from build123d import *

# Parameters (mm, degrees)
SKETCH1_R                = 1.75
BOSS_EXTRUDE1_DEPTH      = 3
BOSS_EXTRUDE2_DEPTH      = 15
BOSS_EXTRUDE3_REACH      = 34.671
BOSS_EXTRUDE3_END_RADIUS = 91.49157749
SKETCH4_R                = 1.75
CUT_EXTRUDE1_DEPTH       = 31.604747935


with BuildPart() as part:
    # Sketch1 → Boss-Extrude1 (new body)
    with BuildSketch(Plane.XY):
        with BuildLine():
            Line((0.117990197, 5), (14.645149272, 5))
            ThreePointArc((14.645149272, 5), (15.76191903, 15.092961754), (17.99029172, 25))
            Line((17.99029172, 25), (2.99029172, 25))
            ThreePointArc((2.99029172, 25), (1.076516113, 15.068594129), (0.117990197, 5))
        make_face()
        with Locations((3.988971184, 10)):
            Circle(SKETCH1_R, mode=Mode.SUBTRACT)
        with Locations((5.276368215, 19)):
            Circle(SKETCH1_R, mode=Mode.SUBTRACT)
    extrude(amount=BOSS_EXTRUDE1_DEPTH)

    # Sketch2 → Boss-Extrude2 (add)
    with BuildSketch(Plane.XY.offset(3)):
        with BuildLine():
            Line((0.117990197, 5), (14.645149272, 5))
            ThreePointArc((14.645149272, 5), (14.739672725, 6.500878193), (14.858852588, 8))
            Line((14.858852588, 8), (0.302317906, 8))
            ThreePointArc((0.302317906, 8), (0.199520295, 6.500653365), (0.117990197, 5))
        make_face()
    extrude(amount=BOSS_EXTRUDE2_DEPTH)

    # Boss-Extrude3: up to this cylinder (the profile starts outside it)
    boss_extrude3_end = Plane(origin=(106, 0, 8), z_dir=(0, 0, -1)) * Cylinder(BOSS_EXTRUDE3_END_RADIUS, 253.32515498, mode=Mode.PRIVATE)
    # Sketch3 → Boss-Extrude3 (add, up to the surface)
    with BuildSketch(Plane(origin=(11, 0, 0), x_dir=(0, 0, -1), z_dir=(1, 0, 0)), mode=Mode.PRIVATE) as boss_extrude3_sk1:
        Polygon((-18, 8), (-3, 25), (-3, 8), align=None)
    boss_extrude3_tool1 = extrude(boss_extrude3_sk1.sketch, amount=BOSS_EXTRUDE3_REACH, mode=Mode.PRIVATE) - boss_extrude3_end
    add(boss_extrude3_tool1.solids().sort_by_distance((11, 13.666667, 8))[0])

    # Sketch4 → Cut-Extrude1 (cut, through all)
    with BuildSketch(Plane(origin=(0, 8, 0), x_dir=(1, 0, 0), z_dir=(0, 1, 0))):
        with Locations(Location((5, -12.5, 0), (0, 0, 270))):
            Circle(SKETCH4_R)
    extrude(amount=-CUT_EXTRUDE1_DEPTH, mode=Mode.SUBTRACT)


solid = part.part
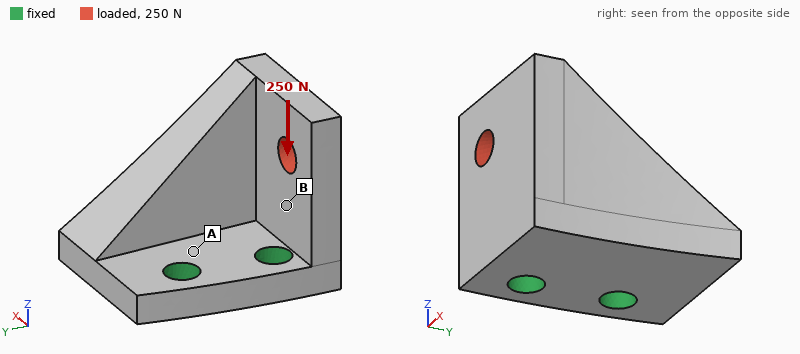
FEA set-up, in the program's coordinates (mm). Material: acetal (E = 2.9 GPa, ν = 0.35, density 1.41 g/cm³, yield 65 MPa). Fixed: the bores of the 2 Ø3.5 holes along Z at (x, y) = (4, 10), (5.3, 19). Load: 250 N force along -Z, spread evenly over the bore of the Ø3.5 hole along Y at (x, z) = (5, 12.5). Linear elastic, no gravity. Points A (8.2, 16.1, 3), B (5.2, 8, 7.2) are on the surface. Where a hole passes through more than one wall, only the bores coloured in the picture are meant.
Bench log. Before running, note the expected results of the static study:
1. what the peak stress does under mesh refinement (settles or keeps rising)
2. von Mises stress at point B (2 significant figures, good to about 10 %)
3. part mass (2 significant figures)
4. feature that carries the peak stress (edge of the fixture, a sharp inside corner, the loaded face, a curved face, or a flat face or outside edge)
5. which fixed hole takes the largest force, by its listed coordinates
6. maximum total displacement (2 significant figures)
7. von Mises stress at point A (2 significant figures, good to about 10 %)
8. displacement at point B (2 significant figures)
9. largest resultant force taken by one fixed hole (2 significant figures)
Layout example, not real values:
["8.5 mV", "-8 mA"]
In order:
["keeps rising", "12 MPa", "2.9 g", "edge of the fixture", "(4, 10)", "0.18 mm", "4.8 MPa", "0.072 mm", "260 N"]
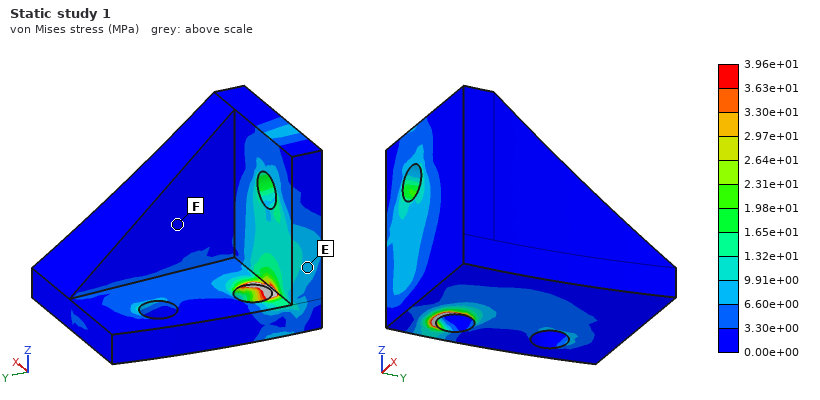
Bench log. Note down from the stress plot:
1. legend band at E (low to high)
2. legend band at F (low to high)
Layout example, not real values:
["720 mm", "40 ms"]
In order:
["6.60e+00 to 9.91e+00 MPa", "0.00e+00 to 3.30e+00 MPa"]
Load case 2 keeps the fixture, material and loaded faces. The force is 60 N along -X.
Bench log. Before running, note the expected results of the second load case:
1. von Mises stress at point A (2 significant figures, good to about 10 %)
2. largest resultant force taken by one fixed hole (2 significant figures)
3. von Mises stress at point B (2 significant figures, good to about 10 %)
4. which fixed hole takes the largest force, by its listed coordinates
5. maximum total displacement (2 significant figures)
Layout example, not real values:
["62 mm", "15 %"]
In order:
["7.7 MPa", "66 N", "5.2 MPa", "(4, 10)", "0.26 mm"]
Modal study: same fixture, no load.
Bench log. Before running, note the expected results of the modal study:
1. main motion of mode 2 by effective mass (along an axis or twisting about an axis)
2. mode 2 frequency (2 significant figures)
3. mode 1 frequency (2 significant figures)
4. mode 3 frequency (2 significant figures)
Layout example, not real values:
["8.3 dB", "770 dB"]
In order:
["along Y", "3500 Hz", "2500 Hz", "6700 Hz"]
